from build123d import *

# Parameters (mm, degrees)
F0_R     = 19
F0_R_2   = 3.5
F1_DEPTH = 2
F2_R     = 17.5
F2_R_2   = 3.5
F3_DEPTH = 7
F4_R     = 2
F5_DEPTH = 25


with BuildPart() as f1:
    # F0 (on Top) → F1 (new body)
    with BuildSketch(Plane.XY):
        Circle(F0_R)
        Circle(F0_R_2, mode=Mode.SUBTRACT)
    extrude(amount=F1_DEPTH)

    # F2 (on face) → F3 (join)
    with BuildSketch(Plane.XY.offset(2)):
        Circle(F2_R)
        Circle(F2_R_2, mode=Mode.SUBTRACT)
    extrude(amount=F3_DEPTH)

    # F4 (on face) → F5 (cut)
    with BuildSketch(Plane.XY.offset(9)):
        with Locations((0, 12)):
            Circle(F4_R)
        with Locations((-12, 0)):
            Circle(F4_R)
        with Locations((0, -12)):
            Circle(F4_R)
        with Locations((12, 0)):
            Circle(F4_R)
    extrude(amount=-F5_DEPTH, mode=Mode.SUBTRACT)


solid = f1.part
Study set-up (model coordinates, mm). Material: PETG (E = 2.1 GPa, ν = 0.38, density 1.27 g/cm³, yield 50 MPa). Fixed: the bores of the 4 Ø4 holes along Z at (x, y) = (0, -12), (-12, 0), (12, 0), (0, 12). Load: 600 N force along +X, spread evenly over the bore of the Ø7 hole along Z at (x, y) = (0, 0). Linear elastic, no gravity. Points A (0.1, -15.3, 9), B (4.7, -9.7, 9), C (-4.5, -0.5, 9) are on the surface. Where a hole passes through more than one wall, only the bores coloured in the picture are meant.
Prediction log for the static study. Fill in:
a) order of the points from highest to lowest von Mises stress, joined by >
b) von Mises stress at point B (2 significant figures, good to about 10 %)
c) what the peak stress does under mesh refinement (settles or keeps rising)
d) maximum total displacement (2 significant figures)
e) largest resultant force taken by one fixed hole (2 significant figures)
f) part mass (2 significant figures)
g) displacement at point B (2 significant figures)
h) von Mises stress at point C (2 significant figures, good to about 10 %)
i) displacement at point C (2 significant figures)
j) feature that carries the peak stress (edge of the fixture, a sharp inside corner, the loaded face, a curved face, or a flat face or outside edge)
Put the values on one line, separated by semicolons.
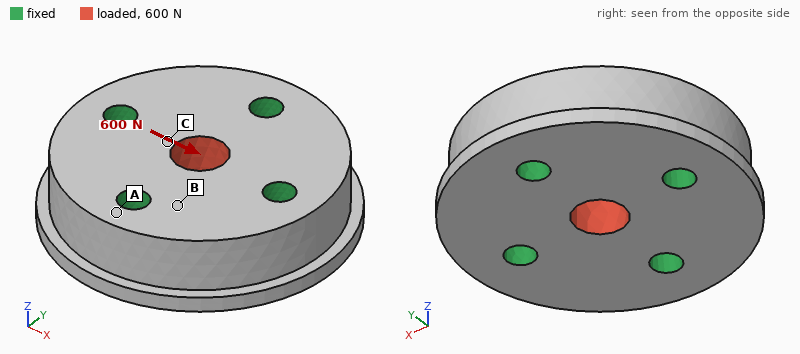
C > B > A; 0.90 MPa; keeps rising; 13 µm; 200 N; 10 g; 3.1 µm; 3.5 MPa; 9.7 µm; edge of the fixture
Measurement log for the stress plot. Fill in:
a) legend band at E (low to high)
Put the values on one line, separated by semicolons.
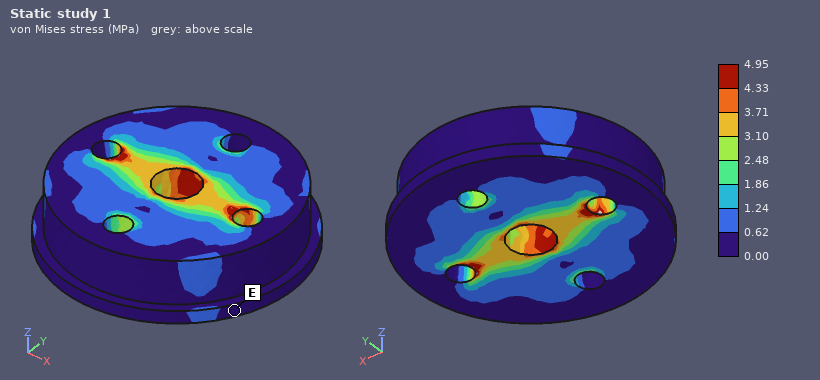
0.00 to 0.62 MPa
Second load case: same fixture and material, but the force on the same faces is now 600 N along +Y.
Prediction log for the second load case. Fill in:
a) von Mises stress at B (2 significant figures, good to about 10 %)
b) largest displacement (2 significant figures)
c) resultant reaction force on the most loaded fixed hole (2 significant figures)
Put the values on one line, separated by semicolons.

1.1 MPa; 13 µm; 200 N
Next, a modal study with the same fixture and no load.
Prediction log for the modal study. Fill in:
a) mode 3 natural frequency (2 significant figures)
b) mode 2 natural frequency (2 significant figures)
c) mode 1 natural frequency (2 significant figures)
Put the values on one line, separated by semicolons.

15 kHz; 15 kHz; 14 kHz
